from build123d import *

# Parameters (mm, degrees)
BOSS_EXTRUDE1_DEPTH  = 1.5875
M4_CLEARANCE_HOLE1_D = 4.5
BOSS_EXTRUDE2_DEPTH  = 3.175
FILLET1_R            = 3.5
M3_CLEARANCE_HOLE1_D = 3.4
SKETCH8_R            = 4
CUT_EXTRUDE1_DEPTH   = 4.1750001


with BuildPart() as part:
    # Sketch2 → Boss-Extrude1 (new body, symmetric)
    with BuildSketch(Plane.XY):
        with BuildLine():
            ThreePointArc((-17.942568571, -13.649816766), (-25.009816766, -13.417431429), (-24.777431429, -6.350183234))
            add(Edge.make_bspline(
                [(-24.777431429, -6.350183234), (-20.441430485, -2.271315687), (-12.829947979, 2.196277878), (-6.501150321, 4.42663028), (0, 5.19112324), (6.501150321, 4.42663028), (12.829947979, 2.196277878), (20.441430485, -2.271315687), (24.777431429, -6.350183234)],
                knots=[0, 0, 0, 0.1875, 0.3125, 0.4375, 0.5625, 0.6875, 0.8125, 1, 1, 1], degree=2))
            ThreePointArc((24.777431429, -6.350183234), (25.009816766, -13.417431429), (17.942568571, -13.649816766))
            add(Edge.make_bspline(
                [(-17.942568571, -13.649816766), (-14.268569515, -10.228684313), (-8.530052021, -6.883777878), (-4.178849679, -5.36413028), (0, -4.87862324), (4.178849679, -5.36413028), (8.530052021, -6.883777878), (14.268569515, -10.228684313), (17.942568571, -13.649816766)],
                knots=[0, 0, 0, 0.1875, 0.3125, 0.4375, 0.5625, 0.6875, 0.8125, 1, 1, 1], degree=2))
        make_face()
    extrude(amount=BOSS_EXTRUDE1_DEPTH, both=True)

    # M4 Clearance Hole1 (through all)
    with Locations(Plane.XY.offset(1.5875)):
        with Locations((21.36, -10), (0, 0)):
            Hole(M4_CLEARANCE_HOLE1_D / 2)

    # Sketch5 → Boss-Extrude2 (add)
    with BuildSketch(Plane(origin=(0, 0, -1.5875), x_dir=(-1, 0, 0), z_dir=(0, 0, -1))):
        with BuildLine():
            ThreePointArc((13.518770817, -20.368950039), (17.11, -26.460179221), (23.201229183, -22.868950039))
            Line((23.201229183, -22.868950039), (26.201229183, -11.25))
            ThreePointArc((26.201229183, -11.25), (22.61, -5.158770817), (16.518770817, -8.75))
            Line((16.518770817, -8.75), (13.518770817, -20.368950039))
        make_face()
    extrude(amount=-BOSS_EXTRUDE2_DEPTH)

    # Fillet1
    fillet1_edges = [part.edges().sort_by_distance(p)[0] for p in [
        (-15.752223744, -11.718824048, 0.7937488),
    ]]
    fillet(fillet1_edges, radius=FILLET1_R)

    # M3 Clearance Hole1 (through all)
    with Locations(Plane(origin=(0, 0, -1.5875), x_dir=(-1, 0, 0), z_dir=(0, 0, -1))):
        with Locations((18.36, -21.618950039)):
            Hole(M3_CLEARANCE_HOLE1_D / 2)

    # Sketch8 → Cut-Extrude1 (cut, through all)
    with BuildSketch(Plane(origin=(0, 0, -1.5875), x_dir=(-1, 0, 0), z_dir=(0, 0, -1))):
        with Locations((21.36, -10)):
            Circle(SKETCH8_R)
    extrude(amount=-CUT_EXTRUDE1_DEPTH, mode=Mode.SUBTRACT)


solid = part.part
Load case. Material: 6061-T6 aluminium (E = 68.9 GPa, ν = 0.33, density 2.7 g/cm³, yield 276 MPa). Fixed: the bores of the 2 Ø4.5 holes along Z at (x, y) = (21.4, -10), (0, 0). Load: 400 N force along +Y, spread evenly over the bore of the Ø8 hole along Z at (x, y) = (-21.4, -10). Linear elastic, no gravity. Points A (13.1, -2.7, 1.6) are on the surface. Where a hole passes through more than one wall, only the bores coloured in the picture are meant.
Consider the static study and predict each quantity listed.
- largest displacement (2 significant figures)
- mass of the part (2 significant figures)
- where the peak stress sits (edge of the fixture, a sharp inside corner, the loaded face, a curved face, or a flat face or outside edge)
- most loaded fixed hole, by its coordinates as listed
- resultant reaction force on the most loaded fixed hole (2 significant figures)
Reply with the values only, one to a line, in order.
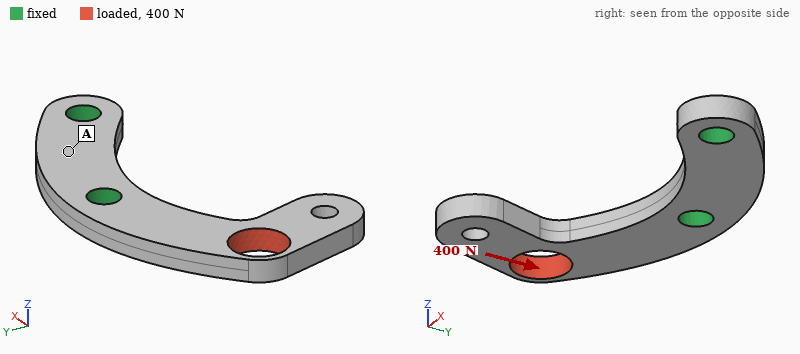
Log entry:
0.23 mm
5.1 g
edge of the fixture
(0, 0)
500 N
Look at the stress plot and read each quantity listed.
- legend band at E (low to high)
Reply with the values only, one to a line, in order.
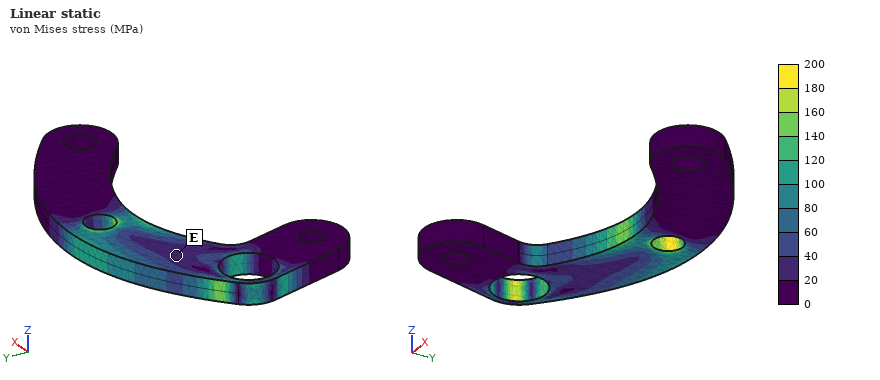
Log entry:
20 to 40 MPa
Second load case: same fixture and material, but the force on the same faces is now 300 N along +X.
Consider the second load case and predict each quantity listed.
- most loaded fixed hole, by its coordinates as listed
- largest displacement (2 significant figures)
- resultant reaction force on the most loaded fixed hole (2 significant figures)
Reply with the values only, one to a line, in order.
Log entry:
(0, 0)
0.11 mm
300 N
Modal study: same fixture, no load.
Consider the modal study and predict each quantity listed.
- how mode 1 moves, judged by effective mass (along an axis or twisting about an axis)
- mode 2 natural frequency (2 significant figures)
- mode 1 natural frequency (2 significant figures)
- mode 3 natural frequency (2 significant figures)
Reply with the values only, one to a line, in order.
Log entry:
along Z
5300 Hz
2300 Hz
6700 Hz
